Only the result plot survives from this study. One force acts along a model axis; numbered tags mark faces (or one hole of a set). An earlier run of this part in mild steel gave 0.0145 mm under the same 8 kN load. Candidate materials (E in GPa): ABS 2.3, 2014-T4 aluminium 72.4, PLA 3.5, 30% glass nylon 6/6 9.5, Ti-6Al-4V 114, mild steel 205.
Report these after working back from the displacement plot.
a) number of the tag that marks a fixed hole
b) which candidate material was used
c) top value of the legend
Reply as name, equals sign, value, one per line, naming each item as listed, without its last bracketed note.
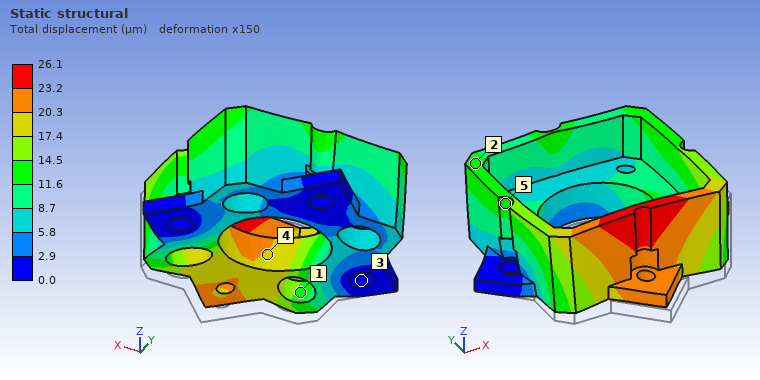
number of the tag that marks a fixed hole = 3
which candidate material was used = Ti-6Al-4V
top value of the legend = 26.1 µm
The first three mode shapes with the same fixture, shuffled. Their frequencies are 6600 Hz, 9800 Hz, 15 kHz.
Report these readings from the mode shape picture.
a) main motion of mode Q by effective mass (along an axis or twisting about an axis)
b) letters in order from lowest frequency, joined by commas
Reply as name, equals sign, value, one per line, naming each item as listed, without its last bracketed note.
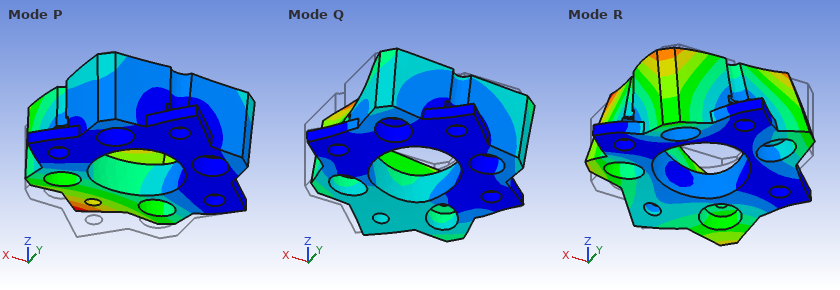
main motion of mode Q by effective mass = along X
letters in order from lowest frequency, joined by commas = P, R, Q
